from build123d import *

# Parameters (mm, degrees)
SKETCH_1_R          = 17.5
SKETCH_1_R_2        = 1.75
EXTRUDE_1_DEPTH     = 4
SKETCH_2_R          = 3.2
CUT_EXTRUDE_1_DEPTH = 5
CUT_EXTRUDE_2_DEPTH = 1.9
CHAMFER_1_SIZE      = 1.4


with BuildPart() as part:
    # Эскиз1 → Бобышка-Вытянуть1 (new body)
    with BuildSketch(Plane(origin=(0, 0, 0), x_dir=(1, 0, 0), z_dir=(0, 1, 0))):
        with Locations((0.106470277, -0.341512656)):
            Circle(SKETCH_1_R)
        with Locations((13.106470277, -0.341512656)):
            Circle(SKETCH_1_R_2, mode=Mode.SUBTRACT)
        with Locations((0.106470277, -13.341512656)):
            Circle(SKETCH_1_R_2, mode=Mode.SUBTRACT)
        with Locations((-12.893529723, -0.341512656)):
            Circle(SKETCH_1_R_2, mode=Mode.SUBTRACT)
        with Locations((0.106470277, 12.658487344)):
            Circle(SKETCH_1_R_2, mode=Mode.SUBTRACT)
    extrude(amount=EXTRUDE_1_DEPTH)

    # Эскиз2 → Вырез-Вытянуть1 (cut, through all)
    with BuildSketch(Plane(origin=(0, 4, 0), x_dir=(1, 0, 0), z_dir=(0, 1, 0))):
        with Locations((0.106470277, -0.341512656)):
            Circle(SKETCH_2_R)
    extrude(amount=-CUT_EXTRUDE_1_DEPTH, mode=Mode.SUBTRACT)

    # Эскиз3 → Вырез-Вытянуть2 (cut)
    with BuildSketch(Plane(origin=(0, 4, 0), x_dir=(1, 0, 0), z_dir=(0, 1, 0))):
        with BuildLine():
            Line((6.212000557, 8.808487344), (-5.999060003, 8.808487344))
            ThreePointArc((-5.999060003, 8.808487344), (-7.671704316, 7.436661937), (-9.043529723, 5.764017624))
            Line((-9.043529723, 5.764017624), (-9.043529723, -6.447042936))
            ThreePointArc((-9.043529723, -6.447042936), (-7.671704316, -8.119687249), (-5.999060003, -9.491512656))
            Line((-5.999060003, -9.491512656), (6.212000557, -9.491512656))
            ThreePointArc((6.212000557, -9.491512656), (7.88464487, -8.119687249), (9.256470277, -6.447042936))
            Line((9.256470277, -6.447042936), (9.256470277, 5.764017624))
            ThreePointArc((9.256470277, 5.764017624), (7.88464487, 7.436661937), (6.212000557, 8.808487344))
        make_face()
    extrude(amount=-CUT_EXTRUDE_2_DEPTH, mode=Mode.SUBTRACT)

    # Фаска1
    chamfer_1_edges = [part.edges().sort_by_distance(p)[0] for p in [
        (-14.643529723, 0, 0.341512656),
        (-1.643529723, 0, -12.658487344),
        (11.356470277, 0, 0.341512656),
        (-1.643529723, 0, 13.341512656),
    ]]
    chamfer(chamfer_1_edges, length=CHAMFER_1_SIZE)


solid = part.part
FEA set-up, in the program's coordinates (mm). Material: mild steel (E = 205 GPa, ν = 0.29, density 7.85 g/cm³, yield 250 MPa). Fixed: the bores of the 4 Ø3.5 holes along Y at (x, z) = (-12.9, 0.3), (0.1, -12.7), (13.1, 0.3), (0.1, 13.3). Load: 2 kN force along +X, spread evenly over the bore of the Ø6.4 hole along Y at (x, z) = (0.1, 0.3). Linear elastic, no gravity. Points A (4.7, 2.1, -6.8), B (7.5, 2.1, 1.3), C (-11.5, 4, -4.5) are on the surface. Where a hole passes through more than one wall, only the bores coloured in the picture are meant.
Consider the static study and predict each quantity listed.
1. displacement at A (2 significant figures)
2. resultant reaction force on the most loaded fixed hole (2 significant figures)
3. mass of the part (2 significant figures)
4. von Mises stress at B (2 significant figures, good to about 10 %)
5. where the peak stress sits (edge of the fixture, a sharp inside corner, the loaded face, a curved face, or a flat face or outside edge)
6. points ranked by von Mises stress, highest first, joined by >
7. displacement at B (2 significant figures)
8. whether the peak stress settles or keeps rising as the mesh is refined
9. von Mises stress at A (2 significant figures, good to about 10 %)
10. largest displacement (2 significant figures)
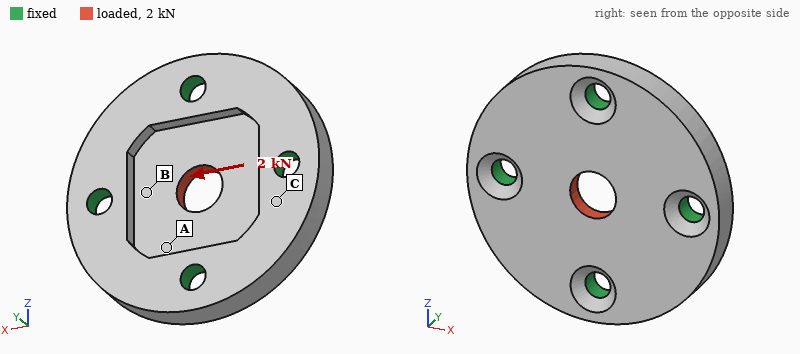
0.85 µm
600 N
23 g
52 MPa
edge of the fixture
B > A > C
1.3 µm
keeps rising
21 MPa
2.3 µm
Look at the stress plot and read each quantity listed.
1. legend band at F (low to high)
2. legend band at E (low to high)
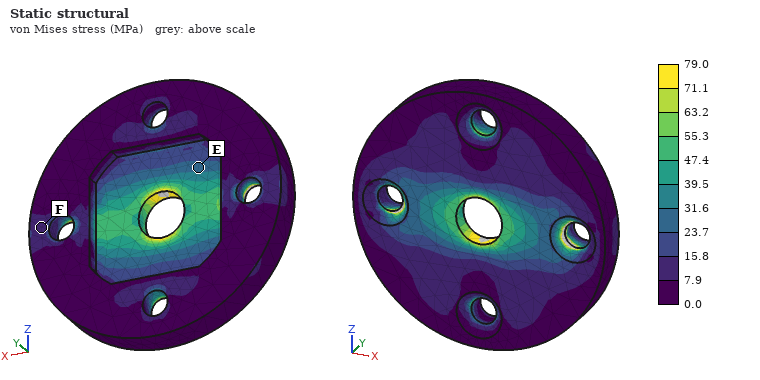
7.9 to 15.8 MPa
23.7 to 31.6 MPa
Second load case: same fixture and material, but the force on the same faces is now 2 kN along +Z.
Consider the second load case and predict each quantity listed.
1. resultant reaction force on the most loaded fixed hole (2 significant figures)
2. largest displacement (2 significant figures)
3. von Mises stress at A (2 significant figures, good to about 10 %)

600 N
2.3 µm
32 MPa
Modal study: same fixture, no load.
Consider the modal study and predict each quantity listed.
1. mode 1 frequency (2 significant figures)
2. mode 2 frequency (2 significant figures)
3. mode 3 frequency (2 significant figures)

31 kHz
33 kHz
33 kHz
